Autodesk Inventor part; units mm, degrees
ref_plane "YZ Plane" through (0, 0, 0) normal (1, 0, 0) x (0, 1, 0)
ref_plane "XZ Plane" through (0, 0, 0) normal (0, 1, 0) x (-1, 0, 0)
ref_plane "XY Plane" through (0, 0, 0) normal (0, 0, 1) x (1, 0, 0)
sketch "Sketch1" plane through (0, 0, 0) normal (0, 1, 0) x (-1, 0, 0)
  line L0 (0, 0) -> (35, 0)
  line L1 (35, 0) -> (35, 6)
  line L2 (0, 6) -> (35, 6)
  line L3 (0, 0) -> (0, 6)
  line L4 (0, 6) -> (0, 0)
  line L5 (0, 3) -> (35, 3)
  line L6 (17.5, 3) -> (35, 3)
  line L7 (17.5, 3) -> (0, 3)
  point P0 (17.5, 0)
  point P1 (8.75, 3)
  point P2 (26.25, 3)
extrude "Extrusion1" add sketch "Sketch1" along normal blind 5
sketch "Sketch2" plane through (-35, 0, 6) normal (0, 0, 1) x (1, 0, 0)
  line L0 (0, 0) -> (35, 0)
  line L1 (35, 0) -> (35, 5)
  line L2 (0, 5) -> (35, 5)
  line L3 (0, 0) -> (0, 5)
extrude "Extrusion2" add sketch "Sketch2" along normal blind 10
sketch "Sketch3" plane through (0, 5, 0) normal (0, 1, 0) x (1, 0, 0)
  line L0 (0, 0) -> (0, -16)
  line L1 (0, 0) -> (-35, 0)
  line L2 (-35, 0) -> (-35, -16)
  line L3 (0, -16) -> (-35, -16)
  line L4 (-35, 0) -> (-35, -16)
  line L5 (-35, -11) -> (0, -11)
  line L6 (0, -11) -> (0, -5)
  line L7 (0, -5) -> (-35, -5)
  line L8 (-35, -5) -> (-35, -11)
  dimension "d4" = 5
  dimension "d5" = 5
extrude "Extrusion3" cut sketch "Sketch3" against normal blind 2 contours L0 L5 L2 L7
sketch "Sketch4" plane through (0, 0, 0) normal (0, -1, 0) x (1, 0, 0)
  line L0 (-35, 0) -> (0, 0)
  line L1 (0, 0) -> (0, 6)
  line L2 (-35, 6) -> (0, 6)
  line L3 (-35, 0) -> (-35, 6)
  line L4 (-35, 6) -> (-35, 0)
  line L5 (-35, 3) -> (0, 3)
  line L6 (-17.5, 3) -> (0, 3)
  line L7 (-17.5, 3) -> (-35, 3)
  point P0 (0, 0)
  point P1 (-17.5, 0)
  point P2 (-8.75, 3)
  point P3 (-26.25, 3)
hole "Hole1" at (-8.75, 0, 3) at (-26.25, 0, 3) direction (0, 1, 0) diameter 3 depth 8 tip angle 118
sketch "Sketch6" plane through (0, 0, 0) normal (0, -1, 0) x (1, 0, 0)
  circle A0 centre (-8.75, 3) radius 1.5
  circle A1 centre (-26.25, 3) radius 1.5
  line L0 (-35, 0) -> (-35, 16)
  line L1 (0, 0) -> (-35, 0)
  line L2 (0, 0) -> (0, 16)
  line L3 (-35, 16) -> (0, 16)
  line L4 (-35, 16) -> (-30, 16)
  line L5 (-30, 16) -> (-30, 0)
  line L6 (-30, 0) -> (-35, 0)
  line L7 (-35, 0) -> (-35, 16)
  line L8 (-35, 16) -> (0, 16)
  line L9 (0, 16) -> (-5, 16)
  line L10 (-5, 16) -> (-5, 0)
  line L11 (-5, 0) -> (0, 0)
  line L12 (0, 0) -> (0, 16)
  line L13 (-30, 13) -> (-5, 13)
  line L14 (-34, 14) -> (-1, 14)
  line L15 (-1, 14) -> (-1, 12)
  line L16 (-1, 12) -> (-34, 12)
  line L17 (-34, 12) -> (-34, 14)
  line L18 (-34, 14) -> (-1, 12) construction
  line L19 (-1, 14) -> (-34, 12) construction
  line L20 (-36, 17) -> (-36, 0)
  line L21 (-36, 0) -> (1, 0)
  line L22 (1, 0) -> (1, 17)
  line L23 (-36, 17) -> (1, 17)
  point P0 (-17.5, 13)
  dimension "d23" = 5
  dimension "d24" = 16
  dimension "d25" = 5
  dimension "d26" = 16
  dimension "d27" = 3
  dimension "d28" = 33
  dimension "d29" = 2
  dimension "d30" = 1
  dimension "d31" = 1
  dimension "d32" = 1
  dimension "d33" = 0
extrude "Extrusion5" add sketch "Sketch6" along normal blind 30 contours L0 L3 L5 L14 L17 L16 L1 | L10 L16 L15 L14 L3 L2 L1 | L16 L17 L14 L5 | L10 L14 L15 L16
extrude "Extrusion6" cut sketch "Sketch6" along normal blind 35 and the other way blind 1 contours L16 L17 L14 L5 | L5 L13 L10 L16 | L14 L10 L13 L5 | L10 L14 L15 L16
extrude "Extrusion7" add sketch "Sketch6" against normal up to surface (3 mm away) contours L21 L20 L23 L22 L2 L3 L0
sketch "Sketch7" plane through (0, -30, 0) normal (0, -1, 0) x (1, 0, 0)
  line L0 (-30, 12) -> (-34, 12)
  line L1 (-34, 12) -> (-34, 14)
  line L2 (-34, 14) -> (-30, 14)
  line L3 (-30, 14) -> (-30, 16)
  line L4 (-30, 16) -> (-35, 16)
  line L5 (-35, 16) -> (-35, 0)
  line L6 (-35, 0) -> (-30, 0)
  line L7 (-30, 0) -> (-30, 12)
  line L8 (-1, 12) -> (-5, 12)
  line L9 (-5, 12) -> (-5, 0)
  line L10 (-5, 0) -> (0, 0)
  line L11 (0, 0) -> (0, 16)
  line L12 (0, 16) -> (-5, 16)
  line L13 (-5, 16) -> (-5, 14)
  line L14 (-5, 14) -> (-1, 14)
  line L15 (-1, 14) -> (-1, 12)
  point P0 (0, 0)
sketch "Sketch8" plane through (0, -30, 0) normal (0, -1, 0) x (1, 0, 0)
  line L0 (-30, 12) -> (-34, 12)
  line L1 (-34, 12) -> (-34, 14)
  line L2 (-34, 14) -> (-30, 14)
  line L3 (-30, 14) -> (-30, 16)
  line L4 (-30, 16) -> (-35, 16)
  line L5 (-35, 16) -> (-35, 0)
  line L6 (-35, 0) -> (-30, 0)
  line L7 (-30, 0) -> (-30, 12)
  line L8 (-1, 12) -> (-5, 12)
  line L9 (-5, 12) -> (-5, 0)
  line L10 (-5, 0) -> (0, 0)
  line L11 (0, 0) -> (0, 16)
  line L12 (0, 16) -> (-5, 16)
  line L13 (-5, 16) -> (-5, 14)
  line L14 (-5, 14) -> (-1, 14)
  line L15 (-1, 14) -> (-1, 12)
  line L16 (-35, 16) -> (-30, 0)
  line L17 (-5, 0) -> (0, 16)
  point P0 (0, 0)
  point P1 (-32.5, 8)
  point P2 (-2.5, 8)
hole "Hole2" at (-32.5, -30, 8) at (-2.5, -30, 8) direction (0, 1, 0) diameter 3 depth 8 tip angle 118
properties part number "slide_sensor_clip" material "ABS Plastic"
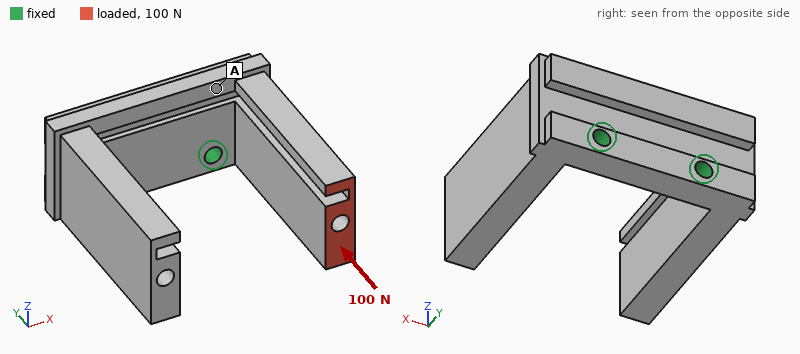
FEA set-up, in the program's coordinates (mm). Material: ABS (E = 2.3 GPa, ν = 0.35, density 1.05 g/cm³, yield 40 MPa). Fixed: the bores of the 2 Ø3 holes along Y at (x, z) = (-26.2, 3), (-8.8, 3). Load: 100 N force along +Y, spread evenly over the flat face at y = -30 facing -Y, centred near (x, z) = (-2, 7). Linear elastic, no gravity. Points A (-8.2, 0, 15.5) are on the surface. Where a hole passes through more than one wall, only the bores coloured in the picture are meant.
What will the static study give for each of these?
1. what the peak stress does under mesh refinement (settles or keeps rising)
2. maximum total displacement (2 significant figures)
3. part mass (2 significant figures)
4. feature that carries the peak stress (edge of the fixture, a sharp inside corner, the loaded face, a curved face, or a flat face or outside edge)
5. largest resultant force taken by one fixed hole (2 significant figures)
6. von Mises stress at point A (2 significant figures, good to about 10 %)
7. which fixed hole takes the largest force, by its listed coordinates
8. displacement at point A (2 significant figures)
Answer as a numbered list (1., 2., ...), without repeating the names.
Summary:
1. keeps rising
2. 0.55 mm
3. 7.0 g
4. edge of the fixture
5. 110 N
6. 2.5 MPa
7. (-8.8, 3)
8. 0.12 mm
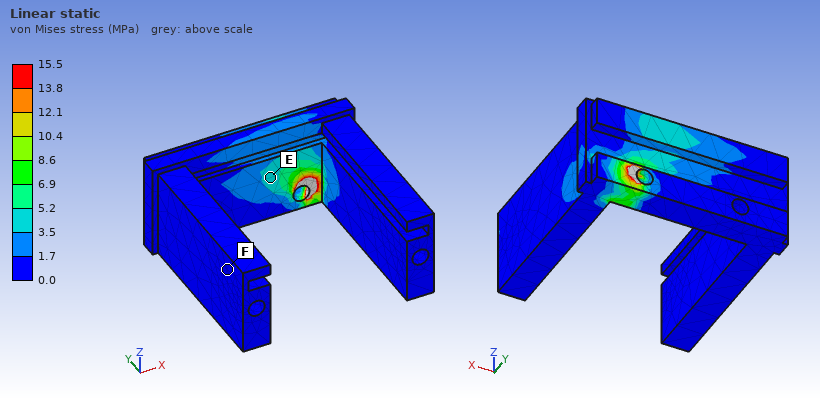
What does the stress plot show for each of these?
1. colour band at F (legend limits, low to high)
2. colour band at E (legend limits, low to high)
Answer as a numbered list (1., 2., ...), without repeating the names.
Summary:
1. 0.0 to 1.7 MPa
2. 3.5 to 5.2 MPa
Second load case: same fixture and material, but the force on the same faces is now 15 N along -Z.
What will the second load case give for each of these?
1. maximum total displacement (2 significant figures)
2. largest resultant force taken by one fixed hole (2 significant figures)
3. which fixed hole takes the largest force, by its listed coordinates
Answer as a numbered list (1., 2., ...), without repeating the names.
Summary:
1. 0.53 mm
2. 20 N
3. (-8.8, 3)
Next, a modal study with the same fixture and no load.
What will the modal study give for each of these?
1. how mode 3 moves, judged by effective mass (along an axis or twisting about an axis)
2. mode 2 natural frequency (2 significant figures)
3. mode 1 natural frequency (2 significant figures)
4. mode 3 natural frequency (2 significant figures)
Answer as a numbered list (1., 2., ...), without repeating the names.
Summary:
1. along Z
2. 840 Hz
3. 820 Hz
4. 1000 Hz
